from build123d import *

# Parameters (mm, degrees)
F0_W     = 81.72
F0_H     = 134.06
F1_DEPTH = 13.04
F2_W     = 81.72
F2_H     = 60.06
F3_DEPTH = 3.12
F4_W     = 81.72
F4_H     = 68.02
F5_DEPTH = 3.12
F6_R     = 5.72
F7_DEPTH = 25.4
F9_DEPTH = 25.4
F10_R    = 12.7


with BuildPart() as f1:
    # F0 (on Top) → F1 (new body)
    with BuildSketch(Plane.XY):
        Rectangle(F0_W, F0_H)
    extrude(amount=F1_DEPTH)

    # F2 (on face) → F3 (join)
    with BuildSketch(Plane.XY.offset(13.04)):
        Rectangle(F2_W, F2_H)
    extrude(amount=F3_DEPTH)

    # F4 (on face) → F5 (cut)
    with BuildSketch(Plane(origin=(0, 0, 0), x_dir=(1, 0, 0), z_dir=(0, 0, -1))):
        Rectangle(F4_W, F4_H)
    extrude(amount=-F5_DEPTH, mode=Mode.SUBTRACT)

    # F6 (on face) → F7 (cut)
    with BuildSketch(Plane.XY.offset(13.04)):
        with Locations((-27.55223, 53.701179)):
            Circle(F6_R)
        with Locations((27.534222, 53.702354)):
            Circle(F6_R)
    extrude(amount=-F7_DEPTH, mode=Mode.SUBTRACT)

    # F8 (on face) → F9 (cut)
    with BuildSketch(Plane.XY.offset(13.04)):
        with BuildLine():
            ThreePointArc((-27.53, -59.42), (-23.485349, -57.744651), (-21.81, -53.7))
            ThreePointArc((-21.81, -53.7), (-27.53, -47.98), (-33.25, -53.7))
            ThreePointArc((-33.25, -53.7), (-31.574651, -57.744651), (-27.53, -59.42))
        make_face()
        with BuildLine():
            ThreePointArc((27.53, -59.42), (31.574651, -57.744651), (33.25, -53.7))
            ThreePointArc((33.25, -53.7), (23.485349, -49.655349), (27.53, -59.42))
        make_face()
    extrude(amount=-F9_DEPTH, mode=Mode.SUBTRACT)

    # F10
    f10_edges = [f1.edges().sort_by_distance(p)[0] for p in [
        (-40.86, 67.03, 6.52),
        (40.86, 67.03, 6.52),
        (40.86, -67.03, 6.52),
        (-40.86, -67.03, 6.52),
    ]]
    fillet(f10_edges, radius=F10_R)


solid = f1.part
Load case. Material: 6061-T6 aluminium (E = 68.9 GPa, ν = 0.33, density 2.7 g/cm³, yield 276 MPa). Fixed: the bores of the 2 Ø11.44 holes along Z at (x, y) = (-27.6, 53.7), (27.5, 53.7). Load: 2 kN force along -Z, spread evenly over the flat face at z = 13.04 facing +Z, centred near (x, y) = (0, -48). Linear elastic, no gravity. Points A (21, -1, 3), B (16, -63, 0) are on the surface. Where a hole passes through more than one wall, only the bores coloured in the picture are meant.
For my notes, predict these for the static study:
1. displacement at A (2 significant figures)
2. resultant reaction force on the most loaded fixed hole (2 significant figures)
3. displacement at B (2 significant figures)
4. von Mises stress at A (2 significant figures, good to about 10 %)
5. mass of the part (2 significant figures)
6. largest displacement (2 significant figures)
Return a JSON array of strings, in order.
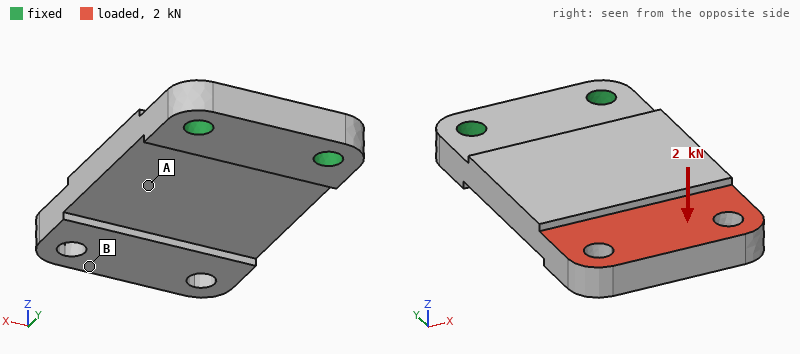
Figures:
["0.29 mm", "1.0 kN", "0.97 mm", "40 MPa", "360 g", "1.0 mm"]
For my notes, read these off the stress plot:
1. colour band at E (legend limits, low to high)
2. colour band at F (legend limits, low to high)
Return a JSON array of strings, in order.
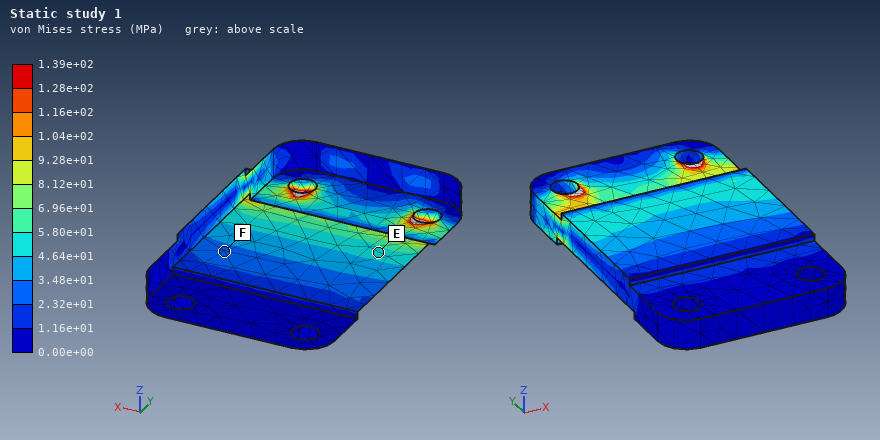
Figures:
["4.64e+01 to 5.80e+01 MPa", "2.32e+01 to 3.48e+01 MPa"]
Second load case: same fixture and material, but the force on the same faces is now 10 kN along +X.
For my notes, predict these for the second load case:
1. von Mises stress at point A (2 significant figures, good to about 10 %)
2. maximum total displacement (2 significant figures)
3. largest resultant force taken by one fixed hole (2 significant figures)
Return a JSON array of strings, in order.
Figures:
["24 MPa", "0.20 mm", "17 kN"]
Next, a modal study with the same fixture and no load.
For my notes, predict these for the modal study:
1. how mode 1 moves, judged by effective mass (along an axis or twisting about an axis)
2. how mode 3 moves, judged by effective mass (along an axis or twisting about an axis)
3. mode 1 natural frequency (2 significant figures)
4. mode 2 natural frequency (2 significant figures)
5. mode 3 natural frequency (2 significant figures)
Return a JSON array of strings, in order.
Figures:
["along Z", "along X", "710 Hz", "2300 Hz", "3600 Hz"]
